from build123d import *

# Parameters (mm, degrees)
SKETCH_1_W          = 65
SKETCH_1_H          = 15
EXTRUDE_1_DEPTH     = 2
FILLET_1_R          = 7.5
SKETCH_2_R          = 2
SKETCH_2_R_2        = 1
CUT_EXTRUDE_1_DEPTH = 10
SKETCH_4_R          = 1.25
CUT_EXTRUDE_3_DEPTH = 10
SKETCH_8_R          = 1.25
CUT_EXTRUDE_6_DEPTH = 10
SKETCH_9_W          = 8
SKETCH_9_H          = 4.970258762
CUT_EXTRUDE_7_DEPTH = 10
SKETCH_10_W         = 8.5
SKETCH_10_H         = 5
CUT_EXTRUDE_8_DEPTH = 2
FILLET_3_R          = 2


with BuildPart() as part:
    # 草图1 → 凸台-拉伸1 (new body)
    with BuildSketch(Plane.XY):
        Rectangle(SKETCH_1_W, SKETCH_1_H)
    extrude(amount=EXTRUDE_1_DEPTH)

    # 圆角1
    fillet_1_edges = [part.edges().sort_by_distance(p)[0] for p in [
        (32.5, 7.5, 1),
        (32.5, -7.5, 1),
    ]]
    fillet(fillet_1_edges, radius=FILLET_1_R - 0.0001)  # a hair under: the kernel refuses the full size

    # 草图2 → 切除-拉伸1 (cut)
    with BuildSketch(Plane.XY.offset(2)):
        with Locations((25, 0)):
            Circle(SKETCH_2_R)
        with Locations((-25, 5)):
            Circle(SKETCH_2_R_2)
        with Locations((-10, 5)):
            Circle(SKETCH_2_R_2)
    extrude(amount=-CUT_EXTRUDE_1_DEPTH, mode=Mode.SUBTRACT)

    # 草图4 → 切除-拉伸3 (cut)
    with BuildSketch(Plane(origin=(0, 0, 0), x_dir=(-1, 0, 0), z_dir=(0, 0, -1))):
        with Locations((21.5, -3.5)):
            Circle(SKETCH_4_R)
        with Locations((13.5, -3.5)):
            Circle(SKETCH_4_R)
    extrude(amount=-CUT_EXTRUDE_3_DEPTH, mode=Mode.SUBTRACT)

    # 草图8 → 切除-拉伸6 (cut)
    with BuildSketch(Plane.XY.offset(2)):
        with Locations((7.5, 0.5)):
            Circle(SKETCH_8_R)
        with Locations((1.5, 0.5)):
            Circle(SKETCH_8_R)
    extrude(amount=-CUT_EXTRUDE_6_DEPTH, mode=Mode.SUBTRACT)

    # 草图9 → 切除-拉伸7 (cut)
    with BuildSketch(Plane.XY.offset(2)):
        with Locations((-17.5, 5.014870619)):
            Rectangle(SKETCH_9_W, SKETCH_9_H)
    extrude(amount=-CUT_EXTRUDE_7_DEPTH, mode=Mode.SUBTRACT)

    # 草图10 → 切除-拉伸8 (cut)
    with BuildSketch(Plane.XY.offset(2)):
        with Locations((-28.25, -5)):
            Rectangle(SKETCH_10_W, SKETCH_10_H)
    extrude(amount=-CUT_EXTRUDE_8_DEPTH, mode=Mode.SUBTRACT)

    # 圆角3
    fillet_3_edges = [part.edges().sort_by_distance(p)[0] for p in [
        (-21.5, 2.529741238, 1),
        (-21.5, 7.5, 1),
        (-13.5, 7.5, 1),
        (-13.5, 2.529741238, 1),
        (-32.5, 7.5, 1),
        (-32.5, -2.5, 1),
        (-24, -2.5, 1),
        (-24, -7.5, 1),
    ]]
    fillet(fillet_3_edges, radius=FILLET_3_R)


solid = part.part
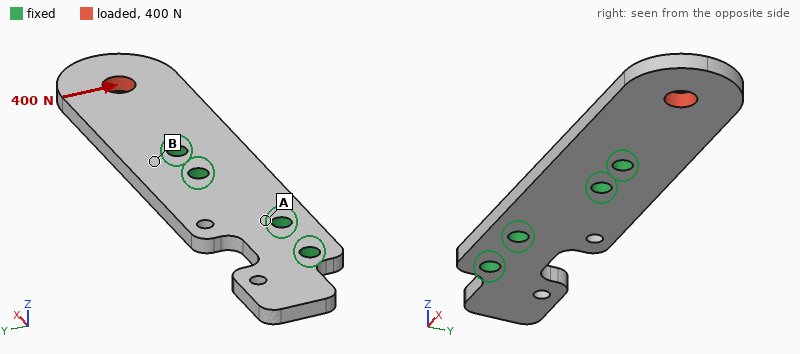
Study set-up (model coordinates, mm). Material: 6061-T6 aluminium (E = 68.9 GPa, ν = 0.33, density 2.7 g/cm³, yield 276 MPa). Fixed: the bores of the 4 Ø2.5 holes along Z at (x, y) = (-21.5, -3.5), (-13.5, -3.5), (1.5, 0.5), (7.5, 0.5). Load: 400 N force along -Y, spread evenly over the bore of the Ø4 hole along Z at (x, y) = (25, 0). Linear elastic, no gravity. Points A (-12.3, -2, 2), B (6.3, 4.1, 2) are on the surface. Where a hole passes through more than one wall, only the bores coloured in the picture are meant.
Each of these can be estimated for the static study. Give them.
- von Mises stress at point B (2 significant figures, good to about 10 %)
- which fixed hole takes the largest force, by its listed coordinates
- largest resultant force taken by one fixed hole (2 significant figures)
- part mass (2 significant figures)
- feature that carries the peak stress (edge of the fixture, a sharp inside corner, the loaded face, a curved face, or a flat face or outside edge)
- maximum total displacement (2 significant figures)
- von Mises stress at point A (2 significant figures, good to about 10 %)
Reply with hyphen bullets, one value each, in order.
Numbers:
- 55 MPa
- (7.5, 0.5)
- 880 N
- 4.5 g
- edge of the fixture
- 74 µm
- 16 MPa
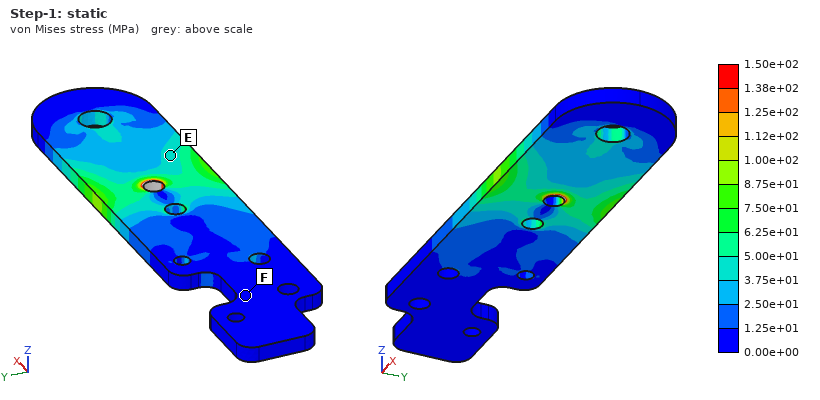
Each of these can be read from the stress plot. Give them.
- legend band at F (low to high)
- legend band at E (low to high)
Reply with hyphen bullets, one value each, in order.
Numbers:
- 0.00e+00 to 1.25e+01 MPa
- 3.75e+01 to 5.00e+01 MPa
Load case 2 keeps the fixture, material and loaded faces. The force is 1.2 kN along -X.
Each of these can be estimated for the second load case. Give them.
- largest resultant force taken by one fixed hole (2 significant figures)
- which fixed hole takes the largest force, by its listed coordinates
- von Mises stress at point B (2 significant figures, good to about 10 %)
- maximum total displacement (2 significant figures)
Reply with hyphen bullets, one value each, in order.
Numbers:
- 840 N
- (7.5, 0.5)
- 24 MPa
- 17 µm
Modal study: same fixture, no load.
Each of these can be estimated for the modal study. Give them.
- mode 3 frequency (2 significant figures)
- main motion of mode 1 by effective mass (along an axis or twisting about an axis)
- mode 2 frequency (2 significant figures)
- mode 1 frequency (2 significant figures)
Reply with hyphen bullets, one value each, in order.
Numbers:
- 9100 Hz
- along Z
- 8800 Hz
- 3100 Hz
